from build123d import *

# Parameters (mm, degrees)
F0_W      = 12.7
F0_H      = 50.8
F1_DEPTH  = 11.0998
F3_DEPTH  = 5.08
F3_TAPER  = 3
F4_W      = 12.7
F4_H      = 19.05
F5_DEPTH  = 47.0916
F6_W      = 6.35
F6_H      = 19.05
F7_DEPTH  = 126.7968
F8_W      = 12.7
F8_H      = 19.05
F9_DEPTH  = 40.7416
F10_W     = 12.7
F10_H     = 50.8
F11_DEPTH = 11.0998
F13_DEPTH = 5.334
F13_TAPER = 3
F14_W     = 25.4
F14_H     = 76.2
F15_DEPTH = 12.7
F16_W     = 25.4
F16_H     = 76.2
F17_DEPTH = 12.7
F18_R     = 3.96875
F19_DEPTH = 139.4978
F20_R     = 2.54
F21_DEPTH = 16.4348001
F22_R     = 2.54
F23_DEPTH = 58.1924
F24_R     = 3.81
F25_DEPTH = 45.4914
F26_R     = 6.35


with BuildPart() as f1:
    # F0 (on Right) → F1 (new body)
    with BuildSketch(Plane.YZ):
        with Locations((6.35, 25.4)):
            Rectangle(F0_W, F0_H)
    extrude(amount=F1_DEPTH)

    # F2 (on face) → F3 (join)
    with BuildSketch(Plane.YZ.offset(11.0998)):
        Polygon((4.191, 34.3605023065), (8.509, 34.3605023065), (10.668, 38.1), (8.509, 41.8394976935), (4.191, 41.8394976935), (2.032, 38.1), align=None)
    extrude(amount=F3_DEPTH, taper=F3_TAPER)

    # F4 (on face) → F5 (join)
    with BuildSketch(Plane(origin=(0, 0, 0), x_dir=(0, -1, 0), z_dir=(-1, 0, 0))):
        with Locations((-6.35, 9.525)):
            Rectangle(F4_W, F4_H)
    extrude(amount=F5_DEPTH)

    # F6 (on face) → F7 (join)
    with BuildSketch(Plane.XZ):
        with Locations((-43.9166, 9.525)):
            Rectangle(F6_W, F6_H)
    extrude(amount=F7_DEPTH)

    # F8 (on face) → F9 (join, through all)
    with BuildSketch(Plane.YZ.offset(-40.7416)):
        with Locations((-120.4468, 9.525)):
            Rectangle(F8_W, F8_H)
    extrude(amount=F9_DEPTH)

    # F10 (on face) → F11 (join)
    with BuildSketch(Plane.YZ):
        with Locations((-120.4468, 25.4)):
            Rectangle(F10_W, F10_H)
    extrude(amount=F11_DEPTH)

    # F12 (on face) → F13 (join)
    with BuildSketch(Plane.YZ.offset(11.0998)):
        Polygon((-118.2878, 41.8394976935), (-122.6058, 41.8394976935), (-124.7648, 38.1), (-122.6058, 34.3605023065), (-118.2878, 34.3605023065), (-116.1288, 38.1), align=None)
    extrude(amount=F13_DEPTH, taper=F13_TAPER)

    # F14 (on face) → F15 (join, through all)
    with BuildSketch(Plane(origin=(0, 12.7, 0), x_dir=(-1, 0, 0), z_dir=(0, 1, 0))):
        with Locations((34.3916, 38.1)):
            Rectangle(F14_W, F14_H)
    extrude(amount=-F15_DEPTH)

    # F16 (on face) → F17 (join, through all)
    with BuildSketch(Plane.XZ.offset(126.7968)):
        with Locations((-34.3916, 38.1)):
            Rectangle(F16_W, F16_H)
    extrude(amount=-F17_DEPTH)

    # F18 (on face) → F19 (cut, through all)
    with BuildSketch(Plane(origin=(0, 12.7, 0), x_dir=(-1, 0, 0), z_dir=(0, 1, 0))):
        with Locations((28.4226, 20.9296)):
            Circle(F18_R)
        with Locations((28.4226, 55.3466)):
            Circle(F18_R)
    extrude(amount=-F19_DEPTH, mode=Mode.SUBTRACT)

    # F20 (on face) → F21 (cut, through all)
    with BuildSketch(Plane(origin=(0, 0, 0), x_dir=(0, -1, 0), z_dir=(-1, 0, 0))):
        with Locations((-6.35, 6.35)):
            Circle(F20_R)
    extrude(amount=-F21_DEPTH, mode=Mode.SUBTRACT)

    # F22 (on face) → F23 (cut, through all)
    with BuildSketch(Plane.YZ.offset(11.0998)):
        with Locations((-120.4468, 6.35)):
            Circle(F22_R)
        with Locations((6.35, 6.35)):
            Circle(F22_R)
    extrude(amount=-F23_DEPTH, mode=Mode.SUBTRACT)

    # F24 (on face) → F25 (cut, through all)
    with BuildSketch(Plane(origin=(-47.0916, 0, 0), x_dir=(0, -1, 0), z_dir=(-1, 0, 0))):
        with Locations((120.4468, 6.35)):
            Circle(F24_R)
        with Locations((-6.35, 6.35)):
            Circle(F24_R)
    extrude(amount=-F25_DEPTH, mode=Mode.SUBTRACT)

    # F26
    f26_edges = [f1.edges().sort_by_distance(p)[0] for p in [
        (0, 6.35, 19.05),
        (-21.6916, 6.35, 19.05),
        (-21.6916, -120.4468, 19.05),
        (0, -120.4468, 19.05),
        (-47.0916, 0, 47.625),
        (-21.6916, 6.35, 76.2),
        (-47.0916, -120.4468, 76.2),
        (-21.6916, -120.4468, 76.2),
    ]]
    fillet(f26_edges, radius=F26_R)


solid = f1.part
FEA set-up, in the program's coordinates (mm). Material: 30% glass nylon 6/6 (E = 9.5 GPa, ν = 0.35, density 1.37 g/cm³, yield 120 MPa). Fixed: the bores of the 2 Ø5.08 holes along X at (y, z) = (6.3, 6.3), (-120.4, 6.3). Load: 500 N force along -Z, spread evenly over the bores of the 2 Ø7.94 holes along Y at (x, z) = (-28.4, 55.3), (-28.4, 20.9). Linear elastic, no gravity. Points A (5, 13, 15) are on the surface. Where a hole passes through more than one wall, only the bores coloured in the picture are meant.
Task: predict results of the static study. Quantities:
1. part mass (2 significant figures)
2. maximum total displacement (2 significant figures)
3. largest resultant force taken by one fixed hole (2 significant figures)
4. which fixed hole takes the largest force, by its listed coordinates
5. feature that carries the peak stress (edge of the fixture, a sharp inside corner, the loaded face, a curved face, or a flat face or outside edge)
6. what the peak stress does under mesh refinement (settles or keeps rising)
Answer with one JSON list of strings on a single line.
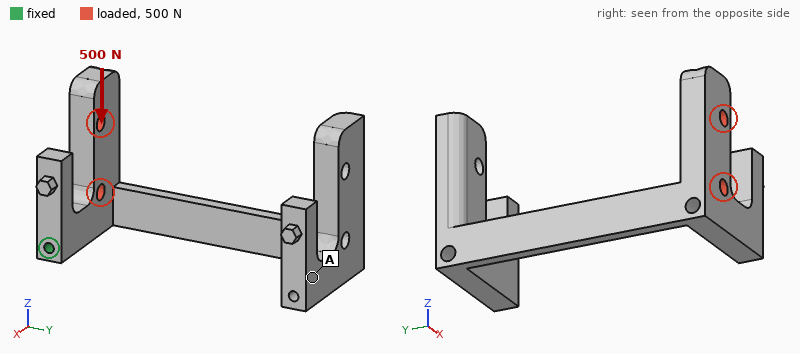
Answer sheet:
["110 g", "0.49 mm", "490 N", "(-120.4, 6.3)", "edge of the fixture", "keeps rising"]
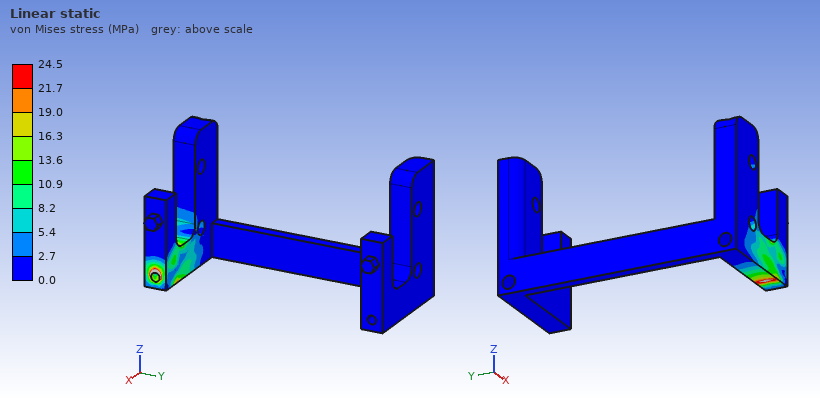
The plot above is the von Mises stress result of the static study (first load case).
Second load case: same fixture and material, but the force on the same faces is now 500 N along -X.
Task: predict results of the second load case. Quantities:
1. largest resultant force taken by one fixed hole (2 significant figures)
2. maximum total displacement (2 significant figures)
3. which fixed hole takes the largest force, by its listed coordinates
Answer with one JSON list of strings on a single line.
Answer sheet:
["500 N", "0.76 mm", "(-120.4, 6.3)"]
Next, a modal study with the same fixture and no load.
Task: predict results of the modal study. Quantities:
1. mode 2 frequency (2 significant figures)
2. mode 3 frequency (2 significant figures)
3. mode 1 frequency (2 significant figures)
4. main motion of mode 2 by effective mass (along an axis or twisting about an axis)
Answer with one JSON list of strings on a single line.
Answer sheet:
["560 Hz", "670 Hz", "350 Hz", "along Y"]
